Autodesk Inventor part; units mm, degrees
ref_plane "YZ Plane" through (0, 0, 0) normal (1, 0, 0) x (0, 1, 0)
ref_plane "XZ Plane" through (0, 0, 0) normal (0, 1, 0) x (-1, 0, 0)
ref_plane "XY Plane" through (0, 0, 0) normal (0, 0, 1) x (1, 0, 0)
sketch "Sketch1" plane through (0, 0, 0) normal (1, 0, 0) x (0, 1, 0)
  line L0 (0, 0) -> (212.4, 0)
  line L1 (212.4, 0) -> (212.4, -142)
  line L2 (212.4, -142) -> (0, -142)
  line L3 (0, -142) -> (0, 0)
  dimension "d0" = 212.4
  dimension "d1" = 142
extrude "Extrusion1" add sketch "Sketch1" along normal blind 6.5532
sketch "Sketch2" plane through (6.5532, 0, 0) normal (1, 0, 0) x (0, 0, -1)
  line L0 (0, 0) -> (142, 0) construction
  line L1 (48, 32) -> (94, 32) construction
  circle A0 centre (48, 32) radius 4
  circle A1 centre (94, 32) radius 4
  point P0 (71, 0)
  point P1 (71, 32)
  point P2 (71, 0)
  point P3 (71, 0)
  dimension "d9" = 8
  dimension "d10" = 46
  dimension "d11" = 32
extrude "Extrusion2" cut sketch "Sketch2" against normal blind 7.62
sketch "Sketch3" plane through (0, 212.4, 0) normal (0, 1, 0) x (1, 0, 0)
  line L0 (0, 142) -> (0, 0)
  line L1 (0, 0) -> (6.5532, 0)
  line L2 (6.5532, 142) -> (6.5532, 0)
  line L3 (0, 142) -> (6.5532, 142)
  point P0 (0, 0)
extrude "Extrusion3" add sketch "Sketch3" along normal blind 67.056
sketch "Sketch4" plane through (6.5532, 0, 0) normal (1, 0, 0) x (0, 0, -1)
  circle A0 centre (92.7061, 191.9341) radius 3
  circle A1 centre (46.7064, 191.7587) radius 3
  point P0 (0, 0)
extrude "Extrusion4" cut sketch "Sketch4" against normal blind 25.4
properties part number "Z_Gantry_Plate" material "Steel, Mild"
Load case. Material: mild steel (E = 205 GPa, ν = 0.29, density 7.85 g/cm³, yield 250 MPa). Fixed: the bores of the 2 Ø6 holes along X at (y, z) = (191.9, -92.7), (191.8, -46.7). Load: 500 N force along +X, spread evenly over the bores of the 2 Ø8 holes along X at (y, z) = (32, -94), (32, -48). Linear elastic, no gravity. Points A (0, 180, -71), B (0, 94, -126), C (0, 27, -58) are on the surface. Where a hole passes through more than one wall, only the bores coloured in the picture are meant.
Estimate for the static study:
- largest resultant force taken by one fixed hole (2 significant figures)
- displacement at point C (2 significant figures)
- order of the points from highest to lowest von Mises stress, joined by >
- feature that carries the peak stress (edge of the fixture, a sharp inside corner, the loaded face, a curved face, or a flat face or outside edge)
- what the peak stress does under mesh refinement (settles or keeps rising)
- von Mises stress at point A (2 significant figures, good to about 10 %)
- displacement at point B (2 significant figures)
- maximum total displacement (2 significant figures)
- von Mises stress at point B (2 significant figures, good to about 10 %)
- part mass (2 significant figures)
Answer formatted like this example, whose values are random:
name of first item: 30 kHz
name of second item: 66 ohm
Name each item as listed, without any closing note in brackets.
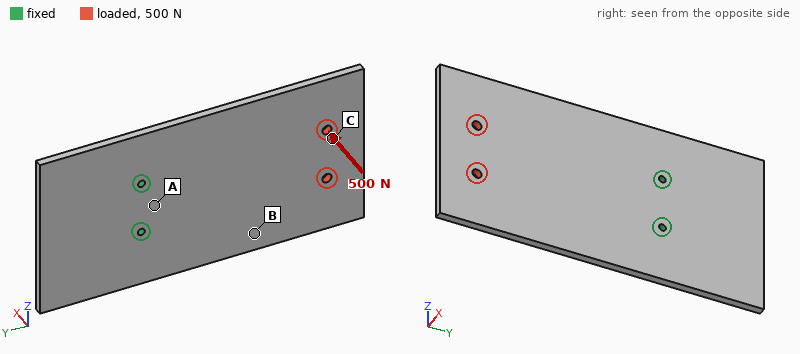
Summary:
largest resultant force taken by one fixed hole: 250 N
displacement at point C: 1.2 mm
order of the points from highest to lowest von Mises stress, joined by >: A > B > C
feature that carries the peak stress: edge of the fixture
what the peak stress does under mesh refinement: keeps rising
von Mises stress at point A: 72 MPa
displacement at point B: 0.50 mm
maximum total displacement: 1.4 mm
von Mises stress at point B: 31 MPa
part mass: 2.0 kg
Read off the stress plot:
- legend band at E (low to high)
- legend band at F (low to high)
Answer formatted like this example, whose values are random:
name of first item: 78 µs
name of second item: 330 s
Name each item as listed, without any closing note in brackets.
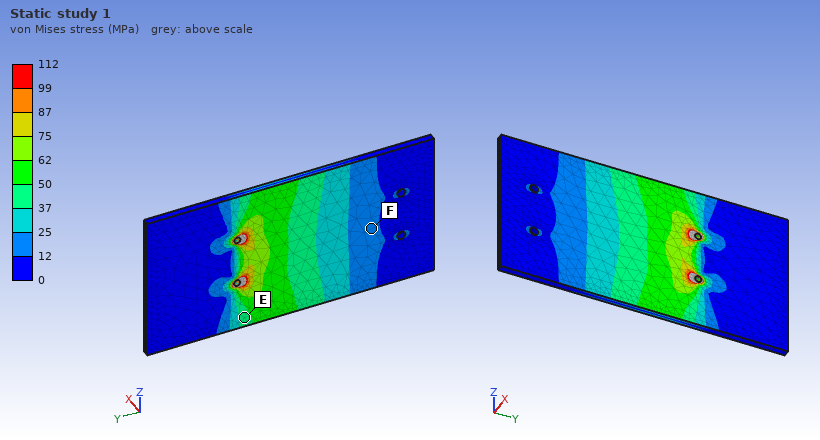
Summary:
legend band at E: 37 to 50 MPa
legend band at F: 12 to 25 MPa
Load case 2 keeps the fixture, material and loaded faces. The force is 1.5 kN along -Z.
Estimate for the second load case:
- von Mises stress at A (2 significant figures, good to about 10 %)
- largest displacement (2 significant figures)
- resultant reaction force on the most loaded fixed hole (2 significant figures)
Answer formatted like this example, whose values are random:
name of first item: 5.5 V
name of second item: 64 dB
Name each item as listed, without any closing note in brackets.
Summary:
von Mises stress at A: 10 MPa
largest displacement: 35 µm
resultant reaction force on the most loaded fixed hole: 5.0 kN
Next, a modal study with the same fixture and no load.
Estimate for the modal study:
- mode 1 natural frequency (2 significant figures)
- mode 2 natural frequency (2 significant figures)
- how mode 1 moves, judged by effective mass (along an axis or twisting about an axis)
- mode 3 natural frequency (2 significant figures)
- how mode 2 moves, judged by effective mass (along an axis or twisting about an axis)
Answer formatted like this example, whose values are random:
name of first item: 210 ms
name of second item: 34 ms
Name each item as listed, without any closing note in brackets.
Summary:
mode 1 natural frequency: 140 Hz
mode 2 natural frequency: 420 Hz
how mode 1 moves, judged by effective mass: along X
mode 3 natural frequency: 610 Hz
how mode 2 moves, judged by effective mass: twisting about Y
